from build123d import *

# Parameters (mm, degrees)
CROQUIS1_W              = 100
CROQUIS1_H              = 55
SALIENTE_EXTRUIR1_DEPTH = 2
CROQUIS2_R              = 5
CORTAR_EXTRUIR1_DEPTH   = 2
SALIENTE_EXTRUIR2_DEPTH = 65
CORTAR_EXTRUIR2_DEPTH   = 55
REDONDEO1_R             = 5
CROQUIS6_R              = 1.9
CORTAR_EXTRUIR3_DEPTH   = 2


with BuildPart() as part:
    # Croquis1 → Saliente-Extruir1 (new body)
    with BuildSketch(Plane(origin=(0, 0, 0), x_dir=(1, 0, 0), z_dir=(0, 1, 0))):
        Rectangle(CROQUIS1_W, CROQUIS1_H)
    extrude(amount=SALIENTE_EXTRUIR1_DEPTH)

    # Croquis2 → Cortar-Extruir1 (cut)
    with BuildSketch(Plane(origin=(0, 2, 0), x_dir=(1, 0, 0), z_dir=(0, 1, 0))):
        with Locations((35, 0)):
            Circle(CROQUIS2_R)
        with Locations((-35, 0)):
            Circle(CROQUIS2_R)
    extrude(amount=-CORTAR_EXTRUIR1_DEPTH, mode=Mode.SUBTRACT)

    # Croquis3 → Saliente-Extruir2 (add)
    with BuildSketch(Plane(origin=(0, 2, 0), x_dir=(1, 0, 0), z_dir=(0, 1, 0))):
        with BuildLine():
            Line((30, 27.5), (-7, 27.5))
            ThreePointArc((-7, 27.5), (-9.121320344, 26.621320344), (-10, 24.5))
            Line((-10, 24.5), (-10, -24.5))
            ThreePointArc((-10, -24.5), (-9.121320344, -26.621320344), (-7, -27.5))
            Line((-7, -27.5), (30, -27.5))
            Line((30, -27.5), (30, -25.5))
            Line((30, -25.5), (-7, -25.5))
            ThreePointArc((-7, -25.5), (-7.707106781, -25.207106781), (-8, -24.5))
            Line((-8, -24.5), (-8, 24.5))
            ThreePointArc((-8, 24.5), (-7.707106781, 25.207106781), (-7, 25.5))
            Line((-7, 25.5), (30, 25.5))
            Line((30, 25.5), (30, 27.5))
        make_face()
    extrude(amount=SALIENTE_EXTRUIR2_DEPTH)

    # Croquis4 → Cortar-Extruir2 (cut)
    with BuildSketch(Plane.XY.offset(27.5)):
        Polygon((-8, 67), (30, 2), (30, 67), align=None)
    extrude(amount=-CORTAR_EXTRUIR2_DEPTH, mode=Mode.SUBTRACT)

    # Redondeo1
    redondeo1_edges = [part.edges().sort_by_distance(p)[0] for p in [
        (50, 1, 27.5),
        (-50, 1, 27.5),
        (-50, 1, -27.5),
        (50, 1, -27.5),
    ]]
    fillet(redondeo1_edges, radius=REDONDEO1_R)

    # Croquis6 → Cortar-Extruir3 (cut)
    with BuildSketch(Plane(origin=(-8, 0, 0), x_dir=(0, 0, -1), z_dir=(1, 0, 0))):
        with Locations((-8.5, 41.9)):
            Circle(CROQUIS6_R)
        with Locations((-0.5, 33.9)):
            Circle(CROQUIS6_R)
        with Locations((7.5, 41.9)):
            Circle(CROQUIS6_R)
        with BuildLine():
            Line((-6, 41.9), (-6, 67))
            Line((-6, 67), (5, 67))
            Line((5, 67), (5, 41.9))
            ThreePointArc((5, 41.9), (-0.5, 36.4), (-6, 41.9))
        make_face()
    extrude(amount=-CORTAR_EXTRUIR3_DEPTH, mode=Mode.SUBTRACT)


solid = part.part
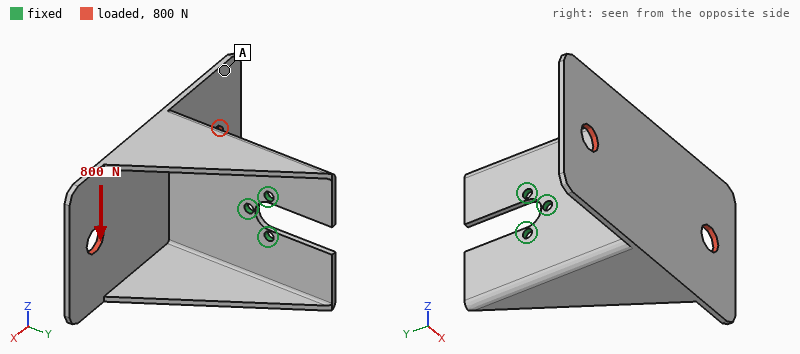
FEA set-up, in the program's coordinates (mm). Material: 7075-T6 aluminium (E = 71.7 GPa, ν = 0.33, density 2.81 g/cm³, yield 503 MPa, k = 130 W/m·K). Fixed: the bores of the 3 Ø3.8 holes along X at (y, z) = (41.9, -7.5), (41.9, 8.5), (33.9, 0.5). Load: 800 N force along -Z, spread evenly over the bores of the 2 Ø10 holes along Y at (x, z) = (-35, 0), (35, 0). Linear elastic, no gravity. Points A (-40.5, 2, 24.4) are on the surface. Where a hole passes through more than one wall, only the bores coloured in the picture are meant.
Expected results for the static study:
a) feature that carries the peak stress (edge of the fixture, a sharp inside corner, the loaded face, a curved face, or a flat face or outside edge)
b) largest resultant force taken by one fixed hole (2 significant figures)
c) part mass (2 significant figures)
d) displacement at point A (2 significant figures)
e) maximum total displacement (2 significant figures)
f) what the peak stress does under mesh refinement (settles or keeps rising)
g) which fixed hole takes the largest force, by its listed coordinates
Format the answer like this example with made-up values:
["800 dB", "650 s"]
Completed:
["edge of the fixture", "1.6 kN", "61 g", "0.85 mm", "1.5 mm", "keeps rising", "(33.9, 0.5)"]
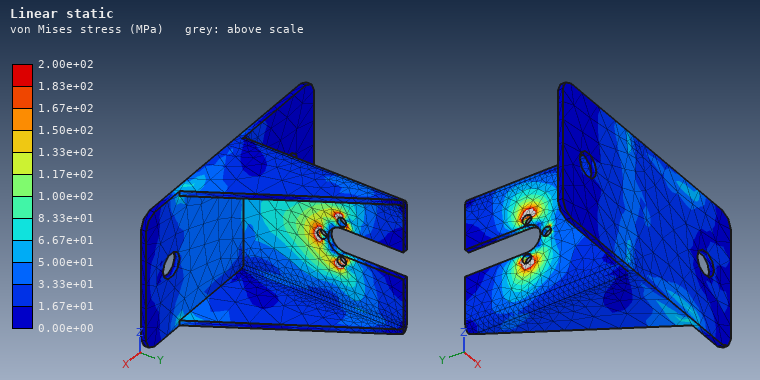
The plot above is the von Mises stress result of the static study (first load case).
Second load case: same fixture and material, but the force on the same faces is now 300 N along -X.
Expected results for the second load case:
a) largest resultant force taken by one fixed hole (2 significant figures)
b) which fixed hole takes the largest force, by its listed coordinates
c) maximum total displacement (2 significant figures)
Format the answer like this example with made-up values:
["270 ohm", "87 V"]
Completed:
["540 N", "(33.9, 0.5)", "1.5 mm"]
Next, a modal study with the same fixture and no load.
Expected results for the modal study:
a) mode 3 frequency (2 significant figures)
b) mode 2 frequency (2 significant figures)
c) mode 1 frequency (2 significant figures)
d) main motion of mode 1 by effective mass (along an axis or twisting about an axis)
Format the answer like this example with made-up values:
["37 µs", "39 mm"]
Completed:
["990 Hz", "420 Hz", "390 Hz", "along X"]
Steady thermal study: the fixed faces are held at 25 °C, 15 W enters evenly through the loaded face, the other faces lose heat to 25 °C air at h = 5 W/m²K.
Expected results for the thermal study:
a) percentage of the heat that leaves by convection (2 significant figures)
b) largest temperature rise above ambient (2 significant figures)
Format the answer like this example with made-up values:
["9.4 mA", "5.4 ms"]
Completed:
["17 %", "43 K"]
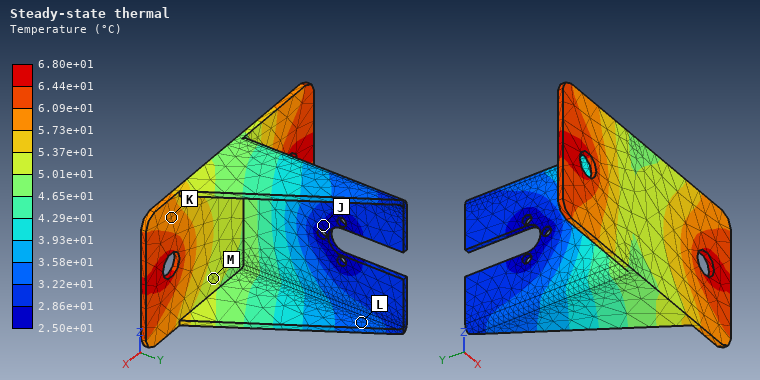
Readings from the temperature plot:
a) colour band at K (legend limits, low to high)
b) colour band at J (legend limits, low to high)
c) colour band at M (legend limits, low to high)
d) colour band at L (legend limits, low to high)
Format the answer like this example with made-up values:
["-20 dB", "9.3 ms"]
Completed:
["5.73e+01 to 6.09e+01 °C", "2.50e+01 to 2.86e+01 °C", "5.01e+01 to 5.37e+01 °C", "3.22e+01 to 3.58e+01 °C"]
